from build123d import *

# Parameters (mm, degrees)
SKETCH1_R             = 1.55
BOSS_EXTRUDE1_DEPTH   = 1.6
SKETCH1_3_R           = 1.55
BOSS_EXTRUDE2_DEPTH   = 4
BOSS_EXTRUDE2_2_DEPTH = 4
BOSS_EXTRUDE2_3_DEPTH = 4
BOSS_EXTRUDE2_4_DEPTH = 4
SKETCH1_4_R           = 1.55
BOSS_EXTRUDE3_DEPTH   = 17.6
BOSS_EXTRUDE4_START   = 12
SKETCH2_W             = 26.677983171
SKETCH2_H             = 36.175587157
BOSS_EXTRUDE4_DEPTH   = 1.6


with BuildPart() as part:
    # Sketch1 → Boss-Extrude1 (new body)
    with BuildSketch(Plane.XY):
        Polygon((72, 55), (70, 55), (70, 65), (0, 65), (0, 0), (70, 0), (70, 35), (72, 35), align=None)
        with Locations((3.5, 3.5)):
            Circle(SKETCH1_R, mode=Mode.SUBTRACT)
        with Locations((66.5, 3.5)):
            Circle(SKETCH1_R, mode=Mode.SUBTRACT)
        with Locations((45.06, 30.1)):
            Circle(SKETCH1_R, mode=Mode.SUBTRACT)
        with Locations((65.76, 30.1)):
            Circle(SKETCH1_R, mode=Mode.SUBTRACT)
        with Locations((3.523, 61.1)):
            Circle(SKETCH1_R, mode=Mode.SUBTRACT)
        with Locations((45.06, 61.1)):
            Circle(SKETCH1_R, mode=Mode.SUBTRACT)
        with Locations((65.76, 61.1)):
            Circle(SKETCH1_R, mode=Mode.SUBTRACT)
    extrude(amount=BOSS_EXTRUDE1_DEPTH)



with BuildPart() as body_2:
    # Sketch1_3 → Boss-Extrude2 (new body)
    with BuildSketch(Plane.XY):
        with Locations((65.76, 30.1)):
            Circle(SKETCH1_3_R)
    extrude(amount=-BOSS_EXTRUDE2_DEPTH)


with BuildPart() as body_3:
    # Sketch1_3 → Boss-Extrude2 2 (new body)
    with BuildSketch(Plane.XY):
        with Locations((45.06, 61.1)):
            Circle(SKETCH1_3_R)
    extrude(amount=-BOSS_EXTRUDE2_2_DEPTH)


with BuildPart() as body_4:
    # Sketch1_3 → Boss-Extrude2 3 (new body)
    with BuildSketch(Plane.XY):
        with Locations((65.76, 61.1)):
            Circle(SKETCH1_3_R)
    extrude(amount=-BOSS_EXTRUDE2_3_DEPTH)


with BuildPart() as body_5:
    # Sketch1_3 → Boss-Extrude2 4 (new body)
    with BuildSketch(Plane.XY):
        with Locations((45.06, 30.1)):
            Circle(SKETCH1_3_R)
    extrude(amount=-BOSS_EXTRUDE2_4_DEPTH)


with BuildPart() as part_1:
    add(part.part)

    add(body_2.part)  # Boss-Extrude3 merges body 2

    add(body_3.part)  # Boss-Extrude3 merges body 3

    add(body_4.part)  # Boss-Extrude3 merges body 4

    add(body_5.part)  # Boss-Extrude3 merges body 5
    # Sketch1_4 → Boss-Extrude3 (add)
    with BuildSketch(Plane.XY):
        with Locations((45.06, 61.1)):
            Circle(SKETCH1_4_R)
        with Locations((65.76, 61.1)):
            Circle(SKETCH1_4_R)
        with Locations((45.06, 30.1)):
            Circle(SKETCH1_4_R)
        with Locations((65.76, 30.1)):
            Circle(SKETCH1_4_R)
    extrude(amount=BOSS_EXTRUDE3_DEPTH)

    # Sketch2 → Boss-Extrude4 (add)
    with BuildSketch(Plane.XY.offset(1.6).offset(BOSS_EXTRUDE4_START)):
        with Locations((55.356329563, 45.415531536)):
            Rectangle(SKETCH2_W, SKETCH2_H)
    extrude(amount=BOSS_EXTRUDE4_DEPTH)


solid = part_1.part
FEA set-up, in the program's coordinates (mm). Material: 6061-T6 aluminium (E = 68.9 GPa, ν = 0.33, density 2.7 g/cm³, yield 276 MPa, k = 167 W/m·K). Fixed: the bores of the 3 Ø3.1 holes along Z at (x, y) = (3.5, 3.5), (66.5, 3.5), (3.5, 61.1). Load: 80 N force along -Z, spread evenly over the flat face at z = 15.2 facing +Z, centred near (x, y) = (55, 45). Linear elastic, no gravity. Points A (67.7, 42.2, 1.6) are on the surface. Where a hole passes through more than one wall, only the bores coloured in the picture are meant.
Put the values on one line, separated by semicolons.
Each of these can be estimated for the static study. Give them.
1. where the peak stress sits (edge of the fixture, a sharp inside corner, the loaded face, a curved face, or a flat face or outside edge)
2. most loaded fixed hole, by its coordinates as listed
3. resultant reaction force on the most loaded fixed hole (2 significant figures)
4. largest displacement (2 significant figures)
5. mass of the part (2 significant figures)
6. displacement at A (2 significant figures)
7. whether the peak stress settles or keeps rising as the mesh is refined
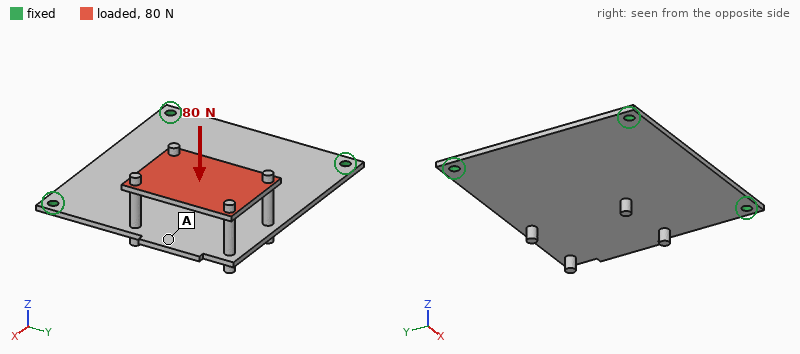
edge of the fixture; (66.5, 3.5); 54 N; 1.2 mm; 25 g; 0.73 mm; keeps rising
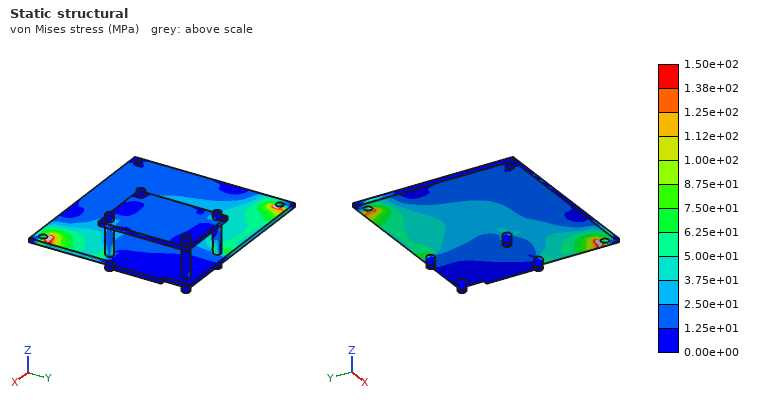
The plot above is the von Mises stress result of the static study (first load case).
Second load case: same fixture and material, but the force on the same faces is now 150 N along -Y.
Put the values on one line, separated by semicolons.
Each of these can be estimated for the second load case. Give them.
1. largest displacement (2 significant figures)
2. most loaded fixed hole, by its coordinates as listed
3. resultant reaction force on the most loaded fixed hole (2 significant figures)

1.0 mm; (66.5, 3.5); 92 N
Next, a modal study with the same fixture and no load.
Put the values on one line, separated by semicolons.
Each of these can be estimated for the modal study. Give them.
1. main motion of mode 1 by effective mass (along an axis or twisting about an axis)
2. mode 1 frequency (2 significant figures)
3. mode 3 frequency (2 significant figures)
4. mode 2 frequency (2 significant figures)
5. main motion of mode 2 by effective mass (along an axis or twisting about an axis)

along Z; 460 Hz; 1700 Hz; 1300 Hz; along Z
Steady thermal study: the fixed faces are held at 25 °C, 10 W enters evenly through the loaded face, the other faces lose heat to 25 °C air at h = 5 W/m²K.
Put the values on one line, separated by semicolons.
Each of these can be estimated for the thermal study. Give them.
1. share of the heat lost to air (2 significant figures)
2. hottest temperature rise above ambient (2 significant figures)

11 %; 55 K
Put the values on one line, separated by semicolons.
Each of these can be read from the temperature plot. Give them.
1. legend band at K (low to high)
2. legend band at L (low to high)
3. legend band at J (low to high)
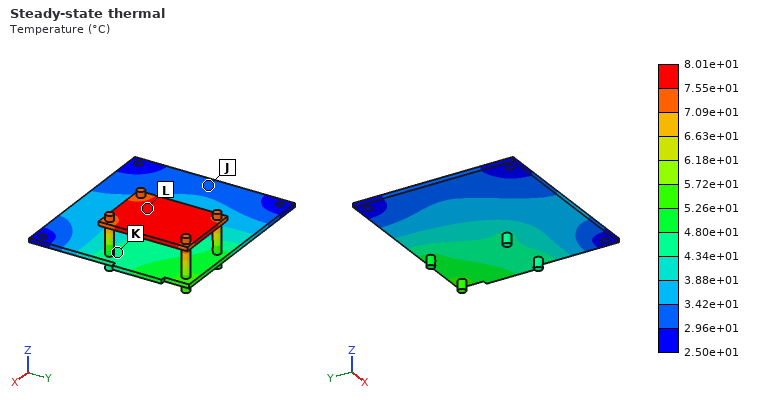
4.34e+01 to 4.80e+01 °C; 7.55e+01 to 8.01e+01 °C; 2.96e+01 to 3.42e+01 °C
